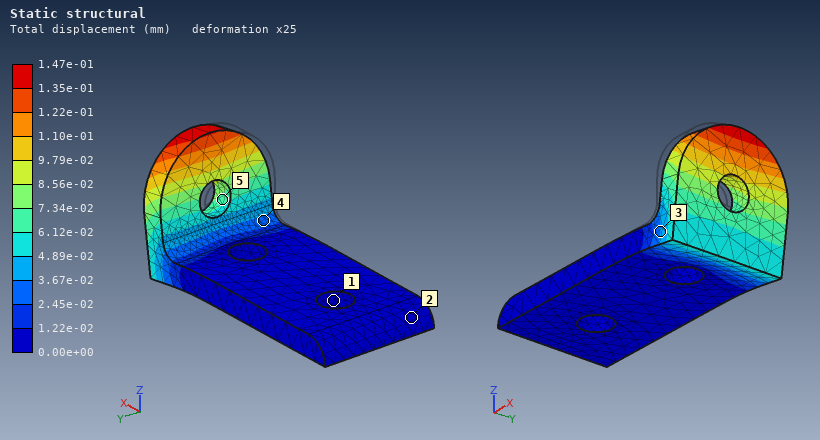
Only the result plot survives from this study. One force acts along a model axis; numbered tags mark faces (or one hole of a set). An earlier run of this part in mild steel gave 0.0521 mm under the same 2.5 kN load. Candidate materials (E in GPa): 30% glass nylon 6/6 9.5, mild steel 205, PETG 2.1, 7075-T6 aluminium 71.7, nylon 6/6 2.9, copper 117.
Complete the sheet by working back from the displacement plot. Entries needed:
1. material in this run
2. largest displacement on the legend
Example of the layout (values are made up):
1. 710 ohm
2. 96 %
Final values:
1. 7075-T6 aluminium
2. 1.47e-01 mm
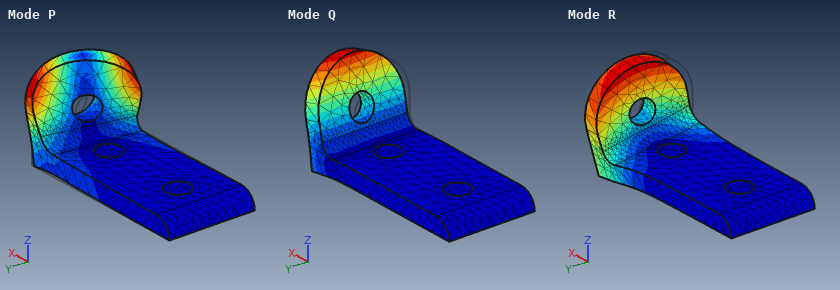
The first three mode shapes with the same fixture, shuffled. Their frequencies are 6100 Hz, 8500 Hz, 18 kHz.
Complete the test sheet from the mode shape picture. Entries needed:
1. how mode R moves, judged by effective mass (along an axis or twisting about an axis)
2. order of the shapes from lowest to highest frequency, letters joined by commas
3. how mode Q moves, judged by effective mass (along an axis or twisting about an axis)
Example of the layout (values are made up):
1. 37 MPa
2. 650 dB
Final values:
1. along Y
2. Q, R, P
3. along X
